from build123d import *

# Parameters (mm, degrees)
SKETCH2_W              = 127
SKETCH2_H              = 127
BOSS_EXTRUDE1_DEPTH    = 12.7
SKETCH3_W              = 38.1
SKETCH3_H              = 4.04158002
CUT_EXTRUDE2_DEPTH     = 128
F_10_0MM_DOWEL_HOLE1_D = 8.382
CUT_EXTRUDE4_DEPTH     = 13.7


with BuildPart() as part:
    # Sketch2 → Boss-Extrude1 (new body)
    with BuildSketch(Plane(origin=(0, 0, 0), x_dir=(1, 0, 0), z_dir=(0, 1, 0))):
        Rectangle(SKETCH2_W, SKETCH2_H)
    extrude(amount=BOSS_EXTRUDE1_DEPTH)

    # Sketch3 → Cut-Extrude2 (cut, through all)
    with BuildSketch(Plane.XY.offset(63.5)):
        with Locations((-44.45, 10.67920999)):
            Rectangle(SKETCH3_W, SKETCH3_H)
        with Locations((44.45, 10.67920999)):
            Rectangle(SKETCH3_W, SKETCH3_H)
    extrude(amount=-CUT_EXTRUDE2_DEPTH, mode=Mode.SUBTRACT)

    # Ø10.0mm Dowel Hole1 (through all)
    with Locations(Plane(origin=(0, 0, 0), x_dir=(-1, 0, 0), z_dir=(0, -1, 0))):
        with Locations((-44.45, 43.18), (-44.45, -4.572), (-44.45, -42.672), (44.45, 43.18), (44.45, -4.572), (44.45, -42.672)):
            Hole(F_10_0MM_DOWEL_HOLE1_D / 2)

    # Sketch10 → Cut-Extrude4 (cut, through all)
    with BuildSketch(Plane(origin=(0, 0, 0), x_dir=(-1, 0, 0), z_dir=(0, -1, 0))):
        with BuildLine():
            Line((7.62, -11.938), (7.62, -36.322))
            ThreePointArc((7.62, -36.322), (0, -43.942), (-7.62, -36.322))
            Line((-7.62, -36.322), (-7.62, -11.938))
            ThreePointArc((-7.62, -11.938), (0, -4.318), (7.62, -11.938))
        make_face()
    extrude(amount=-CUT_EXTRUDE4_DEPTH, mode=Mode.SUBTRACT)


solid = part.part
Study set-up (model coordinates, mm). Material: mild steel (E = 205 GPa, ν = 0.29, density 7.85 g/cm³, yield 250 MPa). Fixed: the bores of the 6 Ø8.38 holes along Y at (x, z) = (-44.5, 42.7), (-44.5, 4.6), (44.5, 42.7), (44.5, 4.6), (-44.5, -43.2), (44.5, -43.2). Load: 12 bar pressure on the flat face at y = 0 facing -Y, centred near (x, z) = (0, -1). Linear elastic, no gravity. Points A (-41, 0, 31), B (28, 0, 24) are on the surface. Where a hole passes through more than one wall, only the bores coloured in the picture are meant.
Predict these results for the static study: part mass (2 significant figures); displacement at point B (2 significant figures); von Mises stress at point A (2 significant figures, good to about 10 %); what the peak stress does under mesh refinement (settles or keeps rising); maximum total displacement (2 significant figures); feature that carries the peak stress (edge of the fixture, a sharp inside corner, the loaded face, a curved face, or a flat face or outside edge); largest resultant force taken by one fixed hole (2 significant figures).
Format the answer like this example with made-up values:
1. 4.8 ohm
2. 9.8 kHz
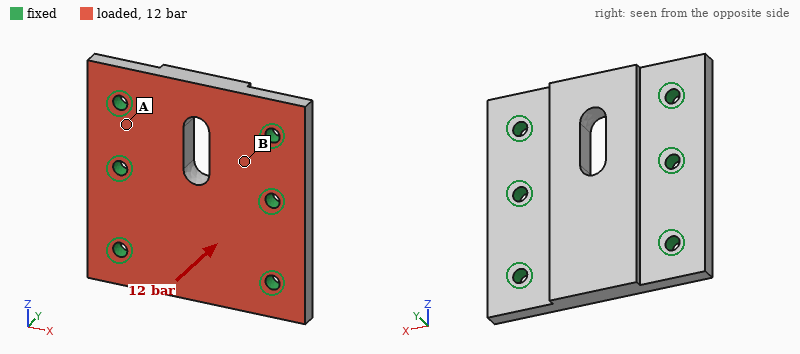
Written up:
1. 1.2 kg
2. 5.7 µm
3. 20 MPa
4. keeps rising
5. 14 µm
6. edge of the fixture
7. 3.5 kN
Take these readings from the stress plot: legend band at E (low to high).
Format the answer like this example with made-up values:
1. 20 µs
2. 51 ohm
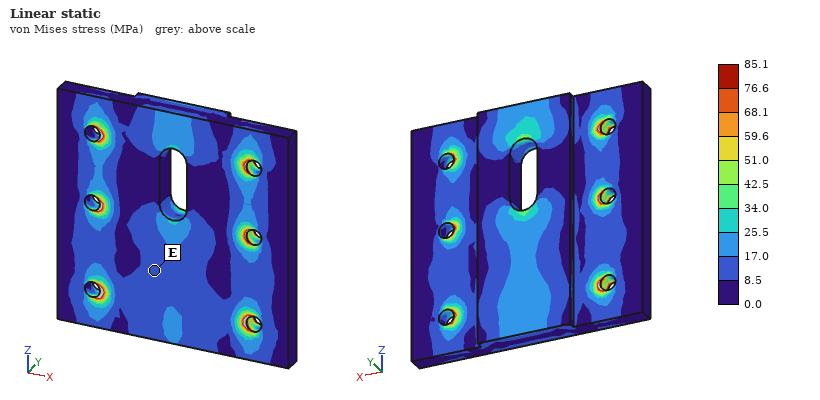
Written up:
1. 8.5 to 17.0 MPa
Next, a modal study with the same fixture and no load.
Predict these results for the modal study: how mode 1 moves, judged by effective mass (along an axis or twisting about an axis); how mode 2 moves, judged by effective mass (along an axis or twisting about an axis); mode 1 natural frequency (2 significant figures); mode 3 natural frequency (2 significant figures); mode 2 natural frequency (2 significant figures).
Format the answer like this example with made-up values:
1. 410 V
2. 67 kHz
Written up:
1. along Y
2. twisting about X
3. 5600 Hz
4. 7800 Hz
5. 5900 Hz
